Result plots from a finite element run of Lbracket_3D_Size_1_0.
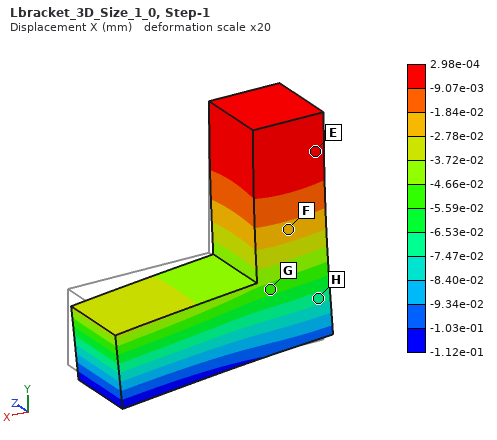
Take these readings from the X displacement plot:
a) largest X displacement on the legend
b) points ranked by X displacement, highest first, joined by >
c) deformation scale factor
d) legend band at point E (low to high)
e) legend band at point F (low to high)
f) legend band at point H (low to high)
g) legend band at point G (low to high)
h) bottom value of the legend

2.98e-04 mm
E > F > G > H
20
-9.07e-03 to 2.98e-04 mm
-2.78e-02 to -1.84e-02 mm
-7.47e-02 to -6.53e-02 mm
-5.59e-02 to -4.66e-02 mm
-1.12e-01 mm
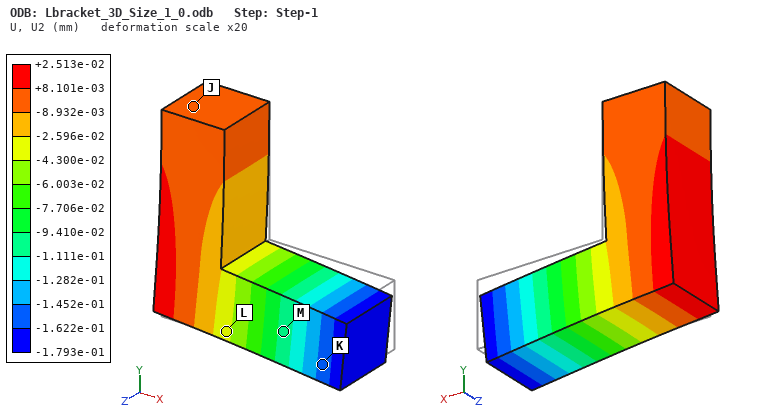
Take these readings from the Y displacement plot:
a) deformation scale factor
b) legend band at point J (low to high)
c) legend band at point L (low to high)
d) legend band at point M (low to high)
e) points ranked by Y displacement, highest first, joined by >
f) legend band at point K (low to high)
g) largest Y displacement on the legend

20
-8.932e-03 to +8.101e-03 mm
-4.300e-02 to -2.596e-02 mm
-1.111e-01 to -9.410e-02 mm
J > L > M > K
-1.622e-01 to -1.452e-01 mm
+2.513e-02 mm
